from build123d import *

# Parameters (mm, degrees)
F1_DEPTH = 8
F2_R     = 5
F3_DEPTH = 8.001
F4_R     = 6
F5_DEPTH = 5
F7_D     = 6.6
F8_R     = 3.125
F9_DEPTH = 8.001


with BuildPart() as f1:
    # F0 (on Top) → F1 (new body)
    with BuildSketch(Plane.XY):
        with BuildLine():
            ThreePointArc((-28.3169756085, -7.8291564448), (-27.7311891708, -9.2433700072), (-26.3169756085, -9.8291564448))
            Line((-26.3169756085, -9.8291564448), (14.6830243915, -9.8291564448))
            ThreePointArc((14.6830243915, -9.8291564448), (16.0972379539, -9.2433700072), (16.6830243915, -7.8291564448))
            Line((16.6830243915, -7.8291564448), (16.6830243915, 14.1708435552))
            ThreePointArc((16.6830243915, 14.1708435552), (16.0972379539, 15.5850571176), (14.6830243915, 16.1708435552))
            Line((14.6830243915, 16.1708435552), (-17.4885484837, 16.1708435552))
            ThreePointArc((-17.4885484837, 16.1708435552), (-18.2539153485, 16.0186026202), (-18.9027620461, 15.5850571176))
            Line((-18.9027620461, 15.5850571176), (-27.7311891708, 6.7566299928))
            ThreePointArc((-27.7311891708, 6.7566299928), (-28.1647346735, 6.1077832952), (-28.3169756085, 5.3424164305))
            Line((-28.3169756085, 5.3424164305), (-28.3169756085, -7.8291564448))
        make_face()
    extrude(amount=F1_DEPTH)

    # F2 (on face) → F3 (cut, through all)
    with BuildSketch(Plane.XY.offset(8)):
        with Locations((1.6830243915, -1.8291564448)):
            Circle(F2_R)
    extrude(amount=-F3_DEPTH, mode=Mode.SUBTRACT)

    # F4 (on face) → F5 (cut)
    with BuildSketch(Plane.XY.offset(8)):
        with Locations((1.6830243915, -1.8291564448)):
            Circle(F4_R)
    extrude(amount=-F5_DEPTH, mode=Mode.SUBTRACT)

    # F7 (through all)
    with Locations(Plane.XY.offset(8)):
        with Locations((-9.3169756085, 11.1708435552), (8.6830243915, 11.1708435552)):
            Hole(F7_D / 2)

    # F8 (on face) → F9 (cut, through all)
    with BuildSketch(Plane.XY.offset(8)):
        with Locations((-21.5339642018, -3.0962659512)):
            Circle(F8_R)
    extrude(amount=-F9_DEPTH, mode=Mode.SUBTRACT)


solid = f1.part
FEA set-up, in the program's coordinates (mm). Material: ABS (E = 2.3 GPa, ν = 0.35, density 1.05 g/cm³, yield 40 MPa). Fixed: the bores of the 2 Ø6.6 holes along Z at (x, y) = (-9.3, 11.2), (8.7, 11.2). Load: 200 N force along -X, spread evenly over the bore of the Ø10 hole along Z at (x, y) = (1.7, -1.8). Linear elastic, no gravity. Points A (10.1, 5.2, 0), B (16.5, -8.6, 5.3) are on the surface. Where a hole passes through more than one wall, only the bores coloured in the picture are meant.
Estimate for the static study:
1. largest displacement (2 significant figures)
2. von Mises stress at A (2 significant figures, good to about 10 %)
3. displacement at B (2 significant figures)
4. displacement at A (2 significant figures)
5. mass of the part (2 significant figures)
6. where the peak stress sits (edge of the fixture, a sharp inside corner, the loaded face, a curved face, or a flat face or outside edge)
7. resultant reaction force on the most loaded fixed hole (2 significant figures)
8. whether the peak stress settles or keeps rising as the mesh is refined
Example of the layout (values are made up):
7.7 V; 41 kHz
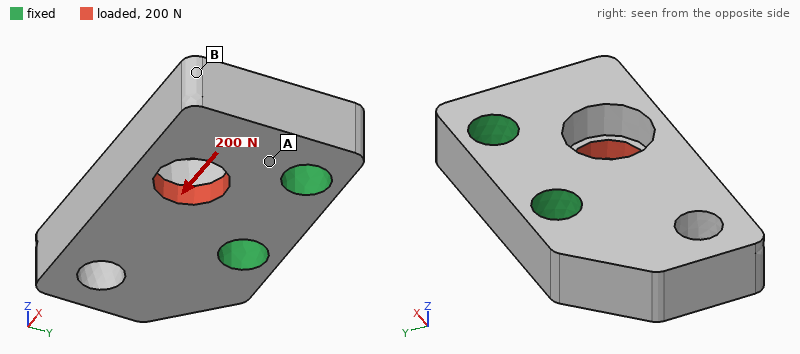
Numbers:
44 µm; 2.2 MPa; 38 µm; 7.2 µm; 7.7 g; a sharp inside corner; 130 N; keeps rising
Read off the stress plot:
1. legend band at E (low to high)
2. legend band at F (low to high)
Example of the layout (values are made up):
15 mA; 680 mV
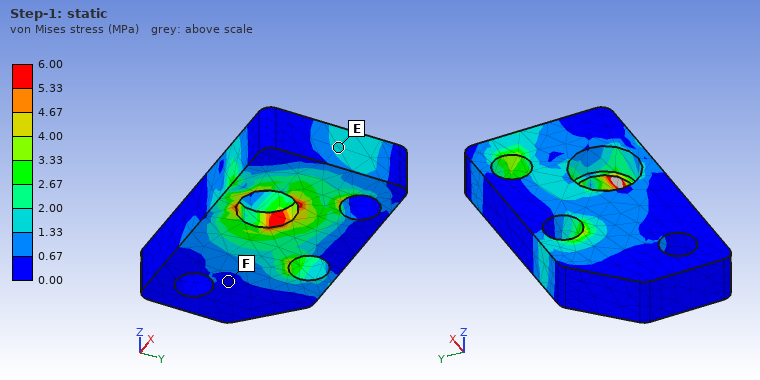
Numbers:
1.33 to 2.00 MPa; 0.00 to 0.67 MPa
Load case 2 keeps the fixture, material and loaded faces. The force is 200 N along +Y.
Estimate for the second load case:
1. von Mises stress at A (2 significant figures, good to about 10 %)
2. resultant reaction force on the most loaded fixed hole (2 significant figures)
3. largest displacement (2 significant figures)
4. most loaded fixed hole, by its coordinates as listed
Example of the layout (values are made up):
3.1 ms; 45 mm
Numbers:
2.7 MPa; 120 N; 44 µm; (8.7, 11.2)
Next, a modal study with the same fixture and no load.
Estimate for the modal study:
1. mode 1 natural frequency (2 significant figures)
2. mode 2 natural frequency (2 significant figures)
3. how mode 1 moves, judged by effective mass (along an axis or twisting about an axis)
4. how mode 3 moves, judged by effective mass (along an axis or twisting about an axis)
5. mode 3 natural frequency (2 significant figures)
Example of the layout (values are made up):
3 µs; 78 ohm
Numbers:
3600 Hz; 4900 Hz; along Z; along X; 5300 Hz
